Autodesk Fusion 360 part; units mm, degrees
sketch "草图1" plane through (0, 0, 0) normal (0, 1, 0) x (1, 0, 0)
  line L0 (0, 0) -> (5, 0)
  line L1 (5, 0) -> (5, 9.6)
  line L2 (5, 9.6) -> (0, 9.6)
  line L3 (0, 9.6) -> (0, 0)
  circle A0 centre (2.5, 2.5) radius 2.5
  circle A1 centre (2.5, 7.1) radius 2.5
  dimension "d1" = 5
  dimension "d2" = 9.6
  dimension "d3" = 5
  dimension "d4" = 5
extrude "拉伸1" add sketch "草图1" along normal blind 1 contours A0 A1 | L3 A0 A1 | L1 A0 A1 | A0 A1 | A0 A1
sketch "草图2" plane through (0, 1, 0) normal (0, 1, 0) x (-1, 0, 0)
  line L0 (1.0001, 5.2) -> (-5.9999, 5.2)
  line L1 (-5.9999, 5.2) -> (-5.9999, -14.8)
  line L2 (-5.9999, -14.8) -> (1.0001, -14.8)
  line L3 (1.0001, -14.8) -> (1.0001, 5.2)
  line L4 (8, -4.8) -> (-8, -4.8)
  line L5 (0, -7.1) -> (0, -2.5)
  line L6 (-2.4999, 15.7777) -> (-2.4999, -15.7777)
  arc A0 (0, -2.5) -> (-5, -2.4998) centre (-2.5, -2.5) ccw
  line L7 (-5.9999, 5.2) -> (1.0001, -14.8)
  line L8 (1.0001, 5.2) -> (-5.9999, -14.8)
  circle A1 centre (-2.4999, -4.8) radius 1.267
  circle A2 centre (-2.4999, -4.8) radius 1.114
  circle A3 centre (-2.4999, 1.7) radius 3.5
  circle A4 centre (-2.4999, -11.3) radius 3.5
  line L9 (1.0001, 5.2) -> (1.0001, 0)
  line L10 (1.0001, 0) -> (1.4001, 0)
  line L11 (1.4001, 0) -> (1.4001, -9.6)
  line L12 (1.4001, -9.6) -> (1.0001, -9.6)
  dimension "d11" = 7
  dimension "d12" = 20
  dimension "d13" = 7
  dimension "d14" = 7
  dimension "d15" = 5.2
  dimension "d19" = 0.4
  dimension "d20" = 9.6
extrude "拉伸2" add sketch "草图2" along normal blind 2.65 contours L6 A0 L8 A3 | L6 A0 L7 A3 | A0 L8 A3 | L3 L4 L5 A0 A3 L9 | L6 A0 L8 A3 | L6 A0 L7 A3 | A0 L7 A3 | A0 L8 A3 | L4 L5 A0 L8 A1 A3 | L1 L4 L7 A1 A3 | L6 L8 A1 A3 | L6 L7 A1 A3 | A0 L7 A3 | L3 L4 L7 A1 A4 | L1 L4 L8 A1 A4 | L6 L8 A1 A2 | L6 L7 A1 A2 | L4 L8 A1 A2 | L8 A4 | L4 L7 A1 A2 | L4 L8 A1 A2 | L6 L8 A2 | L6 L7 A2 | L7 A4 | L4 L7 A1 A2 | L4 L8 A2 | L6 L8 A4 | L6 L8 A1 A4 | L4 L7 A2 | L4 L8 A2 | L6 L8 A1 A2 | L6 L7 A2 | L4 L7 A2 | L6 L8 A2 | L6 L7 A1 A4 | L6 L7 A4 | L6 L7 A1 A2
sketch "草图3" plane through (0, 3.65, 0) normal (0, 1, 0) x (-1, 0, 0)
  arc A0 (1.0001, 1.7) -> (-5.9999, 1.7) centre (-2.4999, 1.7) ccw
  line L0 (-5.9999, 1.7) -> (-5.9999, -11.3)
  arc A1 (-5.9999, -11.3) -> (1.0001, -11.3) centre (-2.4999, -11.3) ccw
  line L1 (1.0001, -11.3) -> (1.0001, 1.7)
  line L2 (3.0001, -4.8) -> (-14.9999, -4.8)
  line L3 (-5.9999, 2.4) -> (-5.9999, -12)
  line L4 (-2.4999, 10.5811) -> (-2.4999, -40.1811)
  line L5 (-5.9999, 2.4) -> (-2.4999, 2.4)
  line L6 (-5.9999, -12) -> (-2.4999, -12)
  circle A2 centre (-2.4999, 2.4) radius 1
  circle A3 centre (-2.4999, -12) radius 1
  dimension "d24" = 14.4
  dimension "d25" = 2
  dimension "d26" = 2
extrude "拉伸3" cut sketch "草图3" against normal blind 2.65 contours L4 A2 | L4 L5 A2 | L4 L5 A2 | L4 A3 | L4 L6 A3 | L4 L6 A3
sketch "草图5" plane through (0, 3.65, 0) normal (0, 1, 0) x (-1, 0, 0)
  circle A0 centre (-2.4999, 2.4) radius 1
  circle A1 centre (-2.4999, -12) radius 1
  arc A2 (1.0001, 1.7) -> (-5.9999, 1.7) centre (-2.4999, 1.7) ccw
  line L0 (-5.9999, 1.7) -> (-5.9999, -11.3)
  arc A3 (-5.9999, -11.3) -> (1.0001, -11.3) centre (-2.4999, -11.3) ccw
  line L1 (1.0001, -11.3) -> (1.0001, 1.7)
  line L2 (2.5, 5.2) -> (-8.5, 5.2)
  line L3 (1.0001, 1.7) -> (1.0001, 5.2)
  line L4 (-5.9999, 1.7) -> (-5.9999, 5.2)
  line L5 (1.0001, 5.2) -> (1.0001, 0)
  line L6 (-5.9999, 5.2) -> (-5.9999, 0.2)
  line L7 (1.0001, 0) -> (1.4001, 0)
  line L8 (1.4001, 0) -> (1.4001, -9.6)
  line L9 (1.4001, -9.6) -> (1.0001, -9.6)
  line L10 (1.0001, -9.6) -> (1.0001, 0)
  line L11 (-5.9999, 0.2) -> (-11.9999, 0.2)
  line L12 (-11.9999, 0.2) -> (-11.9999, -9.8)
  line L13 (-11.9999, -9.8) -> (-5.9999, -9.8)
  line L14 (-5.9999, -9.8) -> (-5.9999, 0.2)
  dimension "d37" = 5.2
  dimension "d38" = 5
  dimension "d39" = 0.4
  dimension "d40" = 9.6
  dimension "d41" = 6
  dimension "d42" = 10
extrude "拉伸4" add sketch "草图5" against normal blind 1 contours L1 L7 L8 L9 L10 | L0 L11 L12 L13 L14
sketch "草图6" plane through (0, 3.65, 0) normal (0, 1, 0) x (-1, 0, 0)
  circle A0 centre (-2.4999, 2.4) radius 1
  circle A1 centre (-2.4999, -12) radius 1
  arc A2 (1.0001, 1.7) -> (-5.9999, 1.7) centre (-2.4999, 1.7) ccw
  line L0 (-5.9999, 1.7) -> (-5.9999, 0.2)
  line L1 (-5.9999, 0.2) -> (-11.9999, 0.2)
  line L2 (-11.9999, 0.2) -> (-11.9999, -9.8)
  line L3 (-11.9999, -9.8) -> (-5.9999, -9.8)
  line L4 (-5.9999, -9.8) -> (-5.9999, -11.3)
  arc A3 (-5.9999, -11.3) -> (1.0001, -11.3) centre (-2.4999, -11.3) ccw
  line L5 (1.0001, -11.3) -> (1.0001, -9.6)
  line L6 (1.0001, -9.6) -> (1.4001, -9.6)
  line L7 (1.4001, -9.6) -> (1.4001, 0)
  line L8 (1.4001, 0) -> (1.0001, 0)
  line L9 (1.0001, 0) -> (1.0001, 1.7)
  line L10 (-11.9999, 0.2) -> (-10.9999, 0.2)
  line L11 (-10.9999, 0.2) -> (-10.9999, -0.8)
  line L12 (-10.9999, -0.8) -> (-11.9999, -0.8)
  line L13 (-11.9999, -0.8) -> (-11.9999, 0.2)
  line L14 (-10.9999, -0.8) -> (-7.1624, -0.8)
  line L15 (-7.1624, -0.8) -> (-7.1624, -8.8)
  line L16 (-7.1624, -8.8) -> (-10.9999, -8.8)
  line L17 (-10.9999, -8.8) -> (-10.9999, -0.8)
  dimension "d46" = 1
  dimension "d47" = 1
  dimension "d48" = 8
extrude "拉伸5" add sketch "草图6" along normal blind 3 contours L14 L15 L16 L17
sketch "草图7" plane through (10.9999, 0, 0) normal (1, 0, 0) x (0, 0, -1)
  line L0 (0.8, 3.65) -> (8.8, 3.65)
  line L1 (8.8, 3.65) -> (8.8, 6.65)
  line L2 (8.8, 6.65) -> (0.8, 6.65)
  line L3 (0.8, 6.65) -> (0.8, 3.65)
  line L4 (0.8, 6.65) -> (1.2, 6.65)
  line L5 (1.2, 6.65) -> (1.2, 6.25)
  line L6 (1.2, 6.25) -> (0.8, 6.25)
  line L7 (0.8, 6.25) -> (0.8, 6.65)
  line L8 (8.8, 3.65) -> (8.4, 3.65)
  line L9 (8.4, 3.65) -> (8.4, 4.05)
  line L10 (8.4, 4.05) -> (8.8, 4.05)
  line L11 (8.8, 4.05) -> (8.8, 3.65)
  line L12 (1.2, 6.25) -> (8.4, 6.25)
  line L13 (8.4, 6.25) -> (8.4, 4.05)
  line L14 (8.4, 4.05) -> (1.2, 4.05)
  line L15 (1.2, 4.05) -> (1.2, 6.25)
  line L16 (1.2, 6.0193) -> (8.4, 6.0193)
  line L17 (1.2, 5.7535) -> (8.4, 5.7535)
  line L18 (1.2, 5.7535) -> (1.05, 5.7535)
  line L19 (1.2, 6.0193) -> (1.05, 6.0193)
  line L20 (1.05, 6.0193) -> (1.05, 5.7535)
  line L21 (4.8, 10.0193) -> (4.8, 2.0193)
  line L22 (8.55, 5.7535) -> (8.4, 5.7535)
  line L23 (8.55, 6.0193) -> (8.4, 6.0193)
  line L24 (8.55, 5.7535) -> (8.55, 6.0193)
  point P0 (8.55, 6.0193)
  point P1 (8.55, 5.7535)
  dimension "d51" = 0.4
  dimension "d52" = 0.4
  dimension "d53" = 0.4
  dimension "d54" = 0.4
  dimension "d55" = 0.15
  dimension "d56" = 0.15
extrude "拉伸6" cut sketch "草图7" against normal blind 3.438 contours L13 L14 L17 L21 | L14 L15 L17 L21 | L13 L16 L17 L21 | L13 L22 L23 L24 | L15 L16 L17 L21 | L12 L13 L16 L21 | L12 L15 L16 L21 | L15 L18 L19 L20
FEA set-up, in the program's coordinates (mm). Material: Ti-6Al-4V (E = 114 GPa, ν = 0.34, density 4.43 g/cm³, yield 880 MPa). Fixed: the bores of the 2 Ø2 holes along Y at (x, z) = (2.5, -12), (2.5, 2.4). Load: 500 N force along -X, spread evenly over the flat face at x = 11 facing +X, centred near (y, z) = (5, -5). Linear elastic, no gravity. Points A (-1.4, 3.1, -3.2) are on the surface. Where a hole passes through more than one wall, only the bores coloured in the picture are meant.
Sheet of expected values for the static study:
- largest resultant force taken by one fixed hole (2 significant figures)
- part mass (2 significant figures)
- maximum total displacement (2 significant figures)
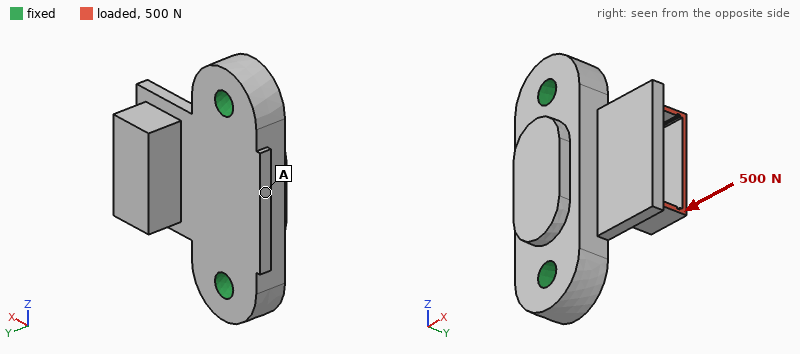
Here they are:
260 N
2.1 g
0.17 mm
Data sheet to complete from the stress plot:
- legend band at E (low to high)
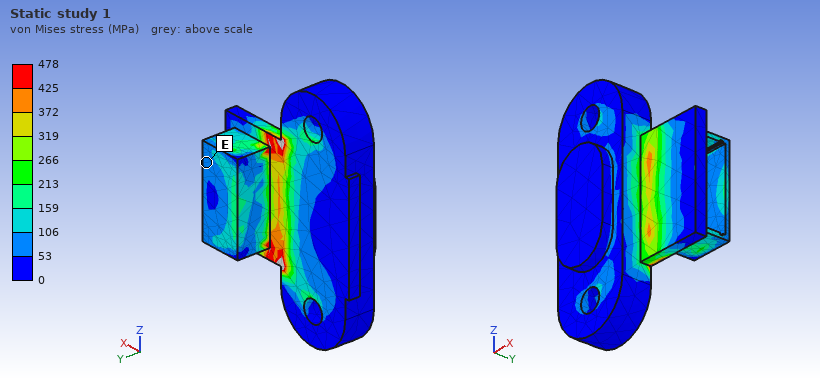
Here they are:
53 to 106 MPa
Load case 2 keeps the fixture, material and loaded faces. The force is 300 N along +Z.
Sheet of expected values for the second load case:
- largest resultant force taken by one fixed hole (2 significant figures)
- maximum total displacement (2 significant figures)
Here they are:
240 N
29 µm
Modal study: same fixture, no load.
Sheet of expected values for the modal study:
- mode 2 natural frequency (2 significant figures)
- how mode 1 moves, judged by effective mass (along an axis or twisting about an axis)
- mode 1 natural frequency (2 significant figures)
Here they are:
33 kHz
along Y
14 kHz
